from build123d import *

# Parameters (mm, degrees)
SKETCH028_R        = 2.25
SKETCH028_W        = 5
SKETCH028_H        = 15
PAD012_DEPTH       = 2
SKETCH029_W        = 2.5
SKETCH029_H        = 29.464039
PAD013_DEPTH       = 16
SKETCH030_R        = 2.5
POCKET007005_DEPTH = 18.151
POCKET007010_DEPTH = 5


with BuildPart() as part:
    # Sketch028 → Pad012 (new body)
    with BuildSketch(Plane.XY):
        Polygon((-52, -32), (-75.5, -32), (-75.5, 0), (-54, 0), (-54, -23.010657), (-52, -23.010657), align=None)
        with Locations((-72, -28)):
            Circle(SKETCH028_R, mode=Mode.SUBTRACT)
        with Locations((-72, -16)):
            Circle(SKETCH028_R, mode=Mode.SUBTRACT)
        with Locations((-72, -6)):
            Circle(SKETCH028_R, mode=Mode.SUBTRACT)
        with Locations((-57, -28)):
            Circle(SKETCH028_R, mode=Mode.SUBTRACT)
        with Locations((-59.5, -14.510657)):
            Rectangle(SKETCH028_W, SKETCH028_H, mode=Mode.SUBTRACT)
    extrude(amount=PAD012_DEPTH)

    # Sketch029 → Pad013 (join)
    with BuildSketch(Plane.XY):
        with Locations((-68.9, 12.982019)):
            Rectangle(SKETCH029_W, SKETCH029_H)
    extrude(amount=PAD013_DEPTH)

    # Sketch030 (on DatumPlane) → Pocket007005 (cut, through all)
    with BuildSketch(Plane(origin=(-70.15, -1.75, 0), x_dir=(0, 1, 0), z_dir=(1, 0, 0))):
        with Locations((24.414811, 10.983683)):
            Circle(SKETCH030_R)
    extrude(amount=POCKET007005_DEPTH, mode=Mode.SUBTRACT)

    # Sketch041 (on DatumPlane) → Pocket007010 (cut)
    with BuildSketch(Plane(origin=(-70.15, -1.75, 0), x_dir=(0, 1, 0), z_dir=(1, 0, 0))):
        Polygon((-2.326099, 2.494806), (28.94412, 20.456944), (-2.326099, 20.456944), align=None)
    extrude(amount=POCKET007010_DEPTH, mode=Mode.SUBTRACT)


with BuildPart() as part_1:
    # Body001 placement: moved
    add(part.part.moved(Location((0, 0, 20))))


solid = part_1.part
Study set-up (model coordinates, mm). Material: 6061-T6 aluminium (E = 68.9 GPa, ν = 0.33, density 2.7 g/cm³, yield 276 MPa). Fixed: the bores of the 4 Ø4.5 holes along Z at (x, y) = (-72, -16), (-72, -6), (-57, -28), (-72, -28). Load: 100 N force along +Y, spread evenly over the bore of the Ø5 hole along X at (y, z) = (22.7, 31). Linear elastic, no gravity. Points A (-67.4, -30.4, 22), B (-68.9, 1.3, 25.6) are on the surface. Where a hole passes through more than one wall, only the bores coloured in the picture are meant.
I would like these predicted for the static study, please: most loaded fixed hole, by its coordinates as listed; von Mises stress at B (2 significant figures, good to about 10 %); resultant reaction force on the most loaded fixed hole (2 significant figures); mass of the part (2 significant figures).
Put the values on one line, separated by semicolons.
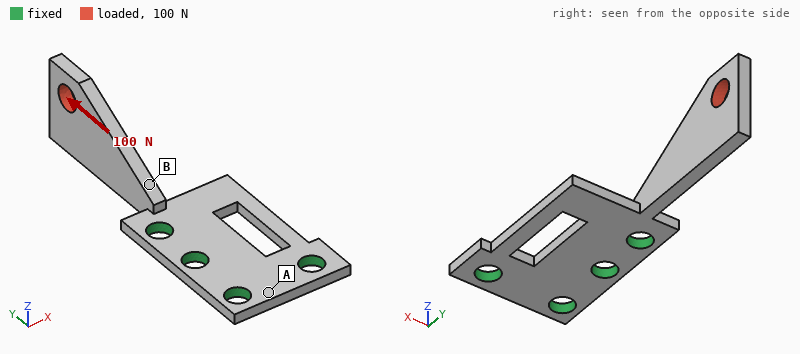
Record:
(-72, -6); 61 MPa; 86 N; 5.2 g
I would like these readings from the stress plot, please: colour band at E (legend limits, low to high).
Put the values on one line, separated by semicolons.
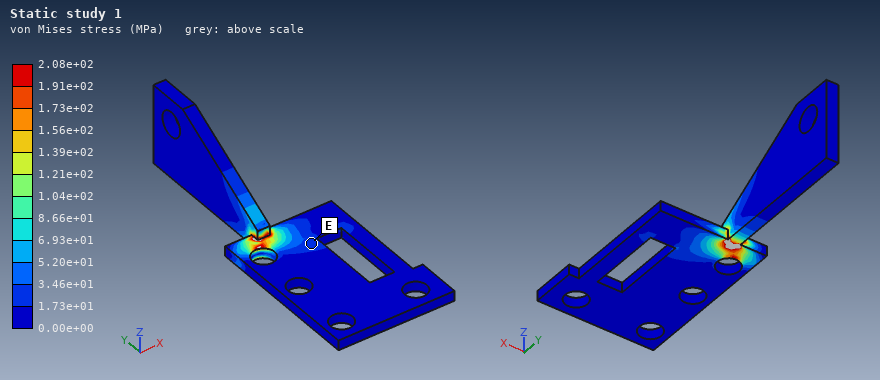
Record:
1.73e+01 to 3.46e+01 MPa
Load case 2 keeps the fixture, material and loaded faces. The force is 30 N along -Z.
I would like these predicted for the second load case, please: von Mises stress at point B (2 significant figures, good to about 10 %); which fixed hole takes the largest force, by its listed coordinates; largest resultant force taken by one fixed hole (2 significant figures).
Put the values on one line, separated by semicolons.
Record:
40 MPa; (-72, -6); 46 N
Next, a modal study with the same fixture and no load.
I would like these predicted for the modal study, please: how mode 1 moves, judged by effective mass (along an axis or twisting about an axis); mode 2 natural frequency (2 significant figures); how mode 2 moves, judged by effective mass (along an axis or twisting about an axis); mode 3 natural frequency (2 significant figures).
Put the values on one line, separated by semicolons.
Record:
along Z; 1400 Hz; along X; 5100 Hz
